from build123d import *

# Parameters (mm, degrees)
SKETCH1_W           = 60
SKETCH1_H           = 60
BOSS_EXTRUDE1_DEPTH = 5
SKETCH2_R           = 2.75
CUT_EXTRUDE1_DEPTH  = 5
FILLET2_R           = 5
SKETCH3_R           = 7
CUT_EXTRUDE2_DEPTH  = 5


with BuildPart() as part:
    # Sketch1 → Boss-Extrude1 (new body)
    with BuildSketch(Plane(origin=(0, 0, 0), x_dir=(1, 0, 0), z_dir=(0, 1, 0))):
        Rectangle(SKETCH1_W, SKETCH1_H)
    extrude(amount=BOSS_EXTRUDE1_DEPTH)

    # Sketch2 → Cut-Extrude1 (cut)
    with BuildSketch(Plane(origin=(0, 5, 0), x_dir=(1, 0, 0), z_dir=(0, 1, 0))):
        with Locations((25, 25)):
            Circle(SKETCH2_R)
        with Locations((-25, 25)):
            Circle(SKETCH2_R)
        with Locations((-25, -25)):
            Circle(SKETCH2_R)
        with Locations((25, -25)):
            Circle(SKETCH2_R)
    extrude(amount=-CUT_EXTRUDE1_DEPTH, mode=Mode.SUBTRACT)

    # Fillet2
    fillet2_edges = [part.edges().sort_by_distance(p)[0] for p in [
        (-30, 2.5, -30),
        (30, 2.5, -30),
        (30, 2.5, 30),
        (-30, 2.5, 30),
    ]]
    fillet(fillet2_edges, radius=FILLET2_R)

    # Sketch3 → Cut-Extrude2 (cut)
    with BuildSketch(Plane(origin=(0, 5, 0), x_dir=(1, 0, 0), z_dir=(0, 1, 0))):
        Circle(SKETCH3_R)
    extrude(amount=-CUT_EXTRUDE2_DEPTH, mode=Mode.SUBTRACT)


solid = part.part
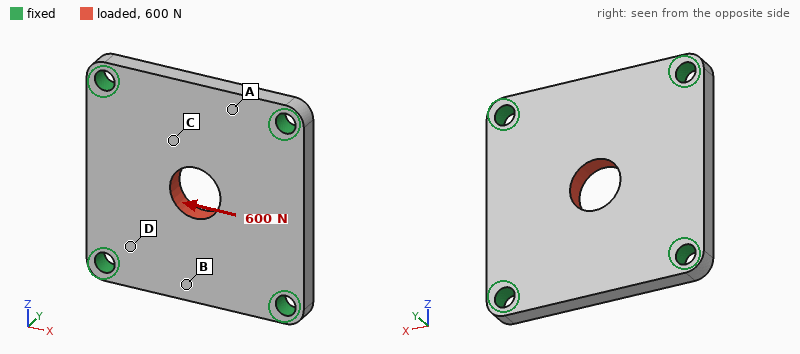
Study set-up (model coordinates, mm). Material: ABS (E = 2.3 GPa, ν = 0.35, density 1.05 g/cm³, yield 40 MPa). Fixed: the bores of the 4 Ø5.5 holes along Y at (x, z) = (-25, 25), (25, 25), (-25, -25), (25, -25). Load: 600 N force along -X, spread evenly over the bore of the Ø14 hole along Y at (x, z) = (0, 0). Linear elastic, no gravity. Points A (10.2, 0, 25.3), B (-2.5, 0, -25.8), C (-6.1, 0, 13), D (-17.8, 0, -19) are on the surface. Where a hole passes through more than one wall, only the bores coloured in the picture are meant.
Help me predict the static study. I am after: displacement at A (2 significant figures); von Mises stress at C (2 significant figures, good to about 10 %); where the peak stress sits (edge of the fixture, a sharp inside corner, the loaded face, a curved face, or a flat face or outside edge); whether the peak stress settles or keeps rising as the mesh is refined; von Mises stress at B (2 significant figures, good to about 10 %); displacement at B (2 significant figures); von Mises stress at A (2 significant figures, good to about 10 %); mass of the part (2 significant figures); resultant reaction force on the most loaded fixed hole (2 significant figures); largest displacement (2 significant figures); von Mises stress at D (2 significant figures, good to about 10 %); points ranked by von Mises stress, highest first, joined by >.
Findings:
8.5 µm
2.0 MPa
edge of the fixture
keeps rising
0.51 MPa
9.7 µm
1.0 MPa
17 g
170 N
39 µm
2.5 MPa
D > C > A > B
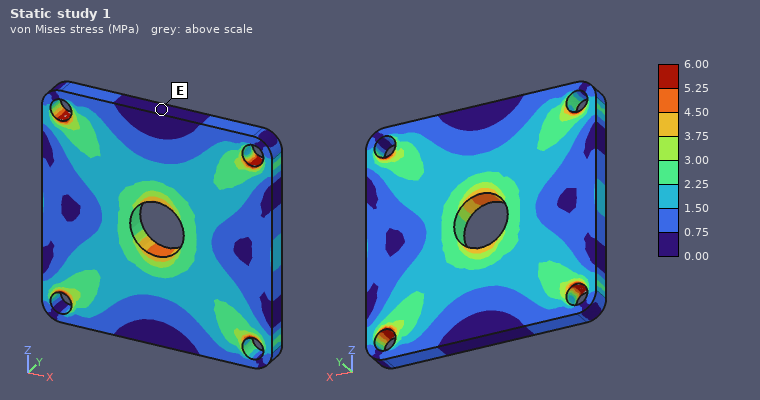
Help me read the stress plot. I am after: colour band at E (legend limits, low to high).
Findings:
0.00 to 0.75 MPa
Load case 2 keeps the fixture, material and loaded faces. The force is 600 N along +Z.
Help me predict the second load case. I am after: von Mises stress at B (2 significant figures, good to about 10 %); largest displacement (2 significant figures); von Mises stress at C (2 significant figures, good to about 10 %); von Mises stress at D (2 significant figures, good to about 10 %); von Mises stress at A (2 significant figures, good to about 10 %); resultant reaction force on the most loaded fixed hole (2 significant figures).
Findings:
0.83 MPa
39 µm
2.0 MPa
2.5 MPa
0.93 MPa
170 N
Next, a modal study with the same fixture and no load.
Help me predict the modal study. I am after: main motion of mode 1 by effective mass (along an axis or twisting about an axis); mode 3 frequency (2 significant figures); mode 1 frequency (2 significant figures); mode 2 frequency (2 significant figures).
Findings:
along Y
3400 Hz
2100 Hz
3400 Hz
